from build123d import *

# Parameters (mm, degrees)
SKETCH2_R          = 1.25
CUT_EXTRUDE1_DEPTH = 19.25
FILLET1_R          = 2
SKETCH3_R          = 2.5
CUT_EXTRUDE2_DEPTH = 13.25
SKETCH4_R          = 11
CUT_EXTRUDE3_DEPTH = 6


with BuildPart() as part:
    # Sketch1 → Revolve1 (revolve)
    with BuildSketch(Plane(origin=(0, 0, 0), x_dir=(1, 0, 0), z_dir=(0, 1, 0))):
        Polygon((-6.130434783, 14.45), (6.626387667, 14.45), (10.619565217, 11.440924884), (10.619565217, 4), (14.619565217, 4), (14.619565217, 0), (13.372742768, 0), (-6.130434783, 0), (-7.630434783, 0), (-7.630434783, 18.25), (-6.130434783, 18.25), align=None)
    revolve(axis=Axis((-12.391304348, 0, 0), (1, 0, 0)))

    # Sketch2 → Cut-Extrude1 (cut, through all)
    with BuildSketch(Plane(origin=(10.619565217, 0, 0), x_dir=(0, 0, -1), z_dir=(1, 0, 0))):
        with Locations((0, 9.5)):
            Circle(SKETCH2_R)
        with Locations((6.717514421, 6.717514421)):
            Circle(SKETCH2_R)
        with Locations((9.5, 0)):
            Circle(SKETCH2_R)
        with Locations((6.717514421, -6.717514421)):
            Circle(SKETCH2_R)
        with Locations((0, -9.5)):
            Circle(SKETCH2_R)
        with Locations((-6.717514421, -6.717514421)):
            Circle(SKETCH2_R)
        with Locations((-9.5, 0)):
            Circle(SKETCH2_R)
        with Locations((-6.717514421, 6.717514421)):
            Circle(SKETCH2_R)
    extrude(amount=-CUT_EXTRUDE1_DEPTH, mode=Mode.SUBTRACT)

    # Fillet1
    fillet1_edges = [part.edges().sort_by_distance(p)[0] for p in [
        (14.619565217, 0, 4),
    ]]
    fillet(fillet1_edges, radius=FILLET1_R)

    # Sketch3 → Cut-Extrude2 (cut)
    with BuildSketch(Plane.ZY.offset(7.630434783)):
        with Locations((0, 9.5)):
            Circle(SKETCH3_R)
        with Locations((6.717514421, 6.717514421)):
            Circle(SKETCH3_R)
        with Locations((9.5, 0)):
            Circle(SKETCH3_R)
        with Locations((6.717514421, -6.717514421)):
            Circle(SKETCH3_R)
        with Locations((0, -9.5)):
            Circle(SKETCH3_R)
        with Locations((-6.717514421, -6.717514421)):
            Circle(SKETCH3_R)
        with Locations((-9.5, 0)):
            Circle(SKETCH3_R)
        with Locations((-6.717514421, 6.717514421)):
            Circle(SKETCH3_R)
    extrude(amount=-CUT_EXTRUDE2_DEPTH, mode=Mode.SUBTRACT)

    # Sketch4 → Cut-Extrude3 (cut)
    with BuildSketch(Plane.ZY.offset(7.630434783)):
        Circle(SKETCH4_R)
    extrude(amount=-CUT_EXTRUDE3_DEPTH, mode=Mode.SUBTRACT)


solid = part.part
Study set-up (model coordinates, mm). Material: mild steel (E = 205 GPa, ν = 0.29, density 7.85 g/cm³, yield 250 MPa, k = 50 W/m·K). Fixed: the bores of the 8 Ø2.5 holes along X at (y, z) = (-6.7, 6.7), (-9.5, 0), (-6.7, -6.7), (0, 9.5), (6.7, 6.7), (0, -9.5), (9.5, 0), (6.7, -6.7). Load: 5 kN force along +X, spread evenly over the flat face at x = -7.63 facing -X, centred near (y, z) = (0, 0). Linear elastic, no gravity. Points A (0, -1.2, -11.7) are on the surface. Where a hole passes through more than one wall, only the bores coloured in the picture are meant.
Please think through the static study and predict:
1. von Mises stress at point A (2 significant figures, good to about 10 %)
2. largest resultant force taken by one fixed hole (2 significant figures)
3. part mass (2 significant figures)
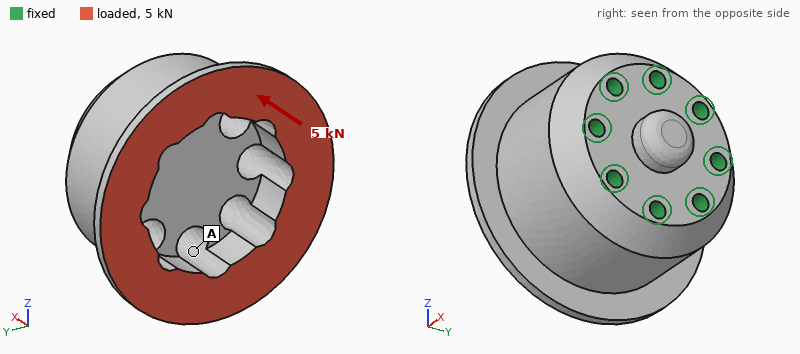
15 MPa
630 N
66 g
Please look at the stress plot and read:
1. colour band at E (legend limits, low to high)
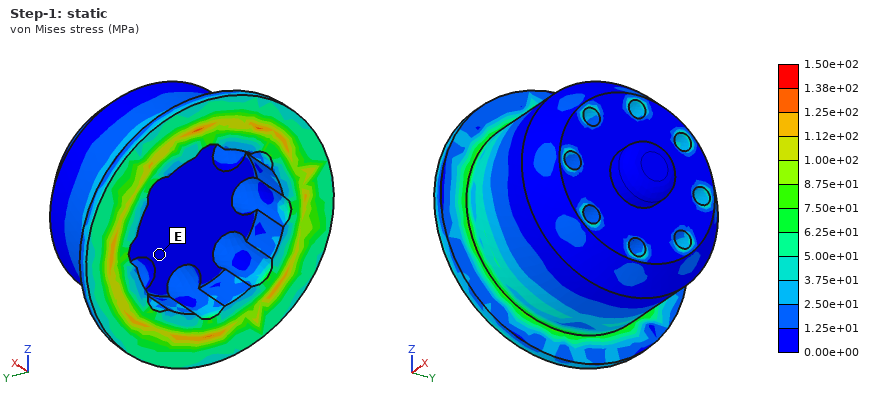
0.00e+00 to 1.25e+01 MPa
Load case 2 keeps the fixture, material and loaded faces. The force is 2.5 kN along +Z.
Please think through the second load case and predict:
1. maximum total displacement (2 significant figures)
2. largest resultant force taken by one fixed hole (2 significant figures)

9.6 µm
860 N
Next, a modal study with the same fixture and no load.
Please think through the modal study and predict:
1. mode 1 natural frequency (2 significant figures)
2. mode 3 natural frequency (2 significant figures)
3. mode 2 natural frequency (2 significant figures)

28 kHz
31 kHz
28 kHz
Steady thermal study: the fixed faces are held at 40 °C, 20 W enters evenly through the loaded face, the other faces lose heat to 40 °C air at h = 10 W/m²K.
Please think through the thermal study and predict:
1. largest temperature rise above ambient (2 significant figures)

25 K
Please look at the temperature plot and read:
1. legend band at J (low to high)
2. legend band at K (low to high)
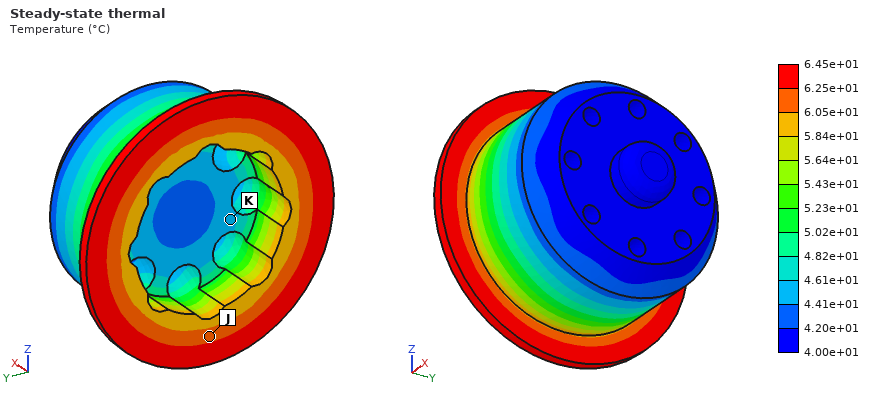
6.05e+01 to 6.25e+01 °C
4.41e+01 to 4.61e+01 °C
